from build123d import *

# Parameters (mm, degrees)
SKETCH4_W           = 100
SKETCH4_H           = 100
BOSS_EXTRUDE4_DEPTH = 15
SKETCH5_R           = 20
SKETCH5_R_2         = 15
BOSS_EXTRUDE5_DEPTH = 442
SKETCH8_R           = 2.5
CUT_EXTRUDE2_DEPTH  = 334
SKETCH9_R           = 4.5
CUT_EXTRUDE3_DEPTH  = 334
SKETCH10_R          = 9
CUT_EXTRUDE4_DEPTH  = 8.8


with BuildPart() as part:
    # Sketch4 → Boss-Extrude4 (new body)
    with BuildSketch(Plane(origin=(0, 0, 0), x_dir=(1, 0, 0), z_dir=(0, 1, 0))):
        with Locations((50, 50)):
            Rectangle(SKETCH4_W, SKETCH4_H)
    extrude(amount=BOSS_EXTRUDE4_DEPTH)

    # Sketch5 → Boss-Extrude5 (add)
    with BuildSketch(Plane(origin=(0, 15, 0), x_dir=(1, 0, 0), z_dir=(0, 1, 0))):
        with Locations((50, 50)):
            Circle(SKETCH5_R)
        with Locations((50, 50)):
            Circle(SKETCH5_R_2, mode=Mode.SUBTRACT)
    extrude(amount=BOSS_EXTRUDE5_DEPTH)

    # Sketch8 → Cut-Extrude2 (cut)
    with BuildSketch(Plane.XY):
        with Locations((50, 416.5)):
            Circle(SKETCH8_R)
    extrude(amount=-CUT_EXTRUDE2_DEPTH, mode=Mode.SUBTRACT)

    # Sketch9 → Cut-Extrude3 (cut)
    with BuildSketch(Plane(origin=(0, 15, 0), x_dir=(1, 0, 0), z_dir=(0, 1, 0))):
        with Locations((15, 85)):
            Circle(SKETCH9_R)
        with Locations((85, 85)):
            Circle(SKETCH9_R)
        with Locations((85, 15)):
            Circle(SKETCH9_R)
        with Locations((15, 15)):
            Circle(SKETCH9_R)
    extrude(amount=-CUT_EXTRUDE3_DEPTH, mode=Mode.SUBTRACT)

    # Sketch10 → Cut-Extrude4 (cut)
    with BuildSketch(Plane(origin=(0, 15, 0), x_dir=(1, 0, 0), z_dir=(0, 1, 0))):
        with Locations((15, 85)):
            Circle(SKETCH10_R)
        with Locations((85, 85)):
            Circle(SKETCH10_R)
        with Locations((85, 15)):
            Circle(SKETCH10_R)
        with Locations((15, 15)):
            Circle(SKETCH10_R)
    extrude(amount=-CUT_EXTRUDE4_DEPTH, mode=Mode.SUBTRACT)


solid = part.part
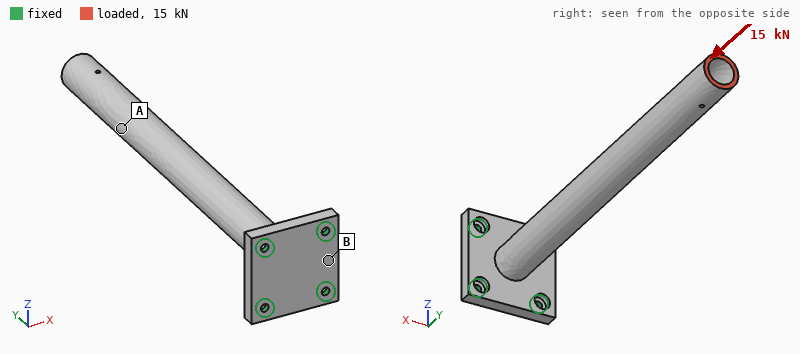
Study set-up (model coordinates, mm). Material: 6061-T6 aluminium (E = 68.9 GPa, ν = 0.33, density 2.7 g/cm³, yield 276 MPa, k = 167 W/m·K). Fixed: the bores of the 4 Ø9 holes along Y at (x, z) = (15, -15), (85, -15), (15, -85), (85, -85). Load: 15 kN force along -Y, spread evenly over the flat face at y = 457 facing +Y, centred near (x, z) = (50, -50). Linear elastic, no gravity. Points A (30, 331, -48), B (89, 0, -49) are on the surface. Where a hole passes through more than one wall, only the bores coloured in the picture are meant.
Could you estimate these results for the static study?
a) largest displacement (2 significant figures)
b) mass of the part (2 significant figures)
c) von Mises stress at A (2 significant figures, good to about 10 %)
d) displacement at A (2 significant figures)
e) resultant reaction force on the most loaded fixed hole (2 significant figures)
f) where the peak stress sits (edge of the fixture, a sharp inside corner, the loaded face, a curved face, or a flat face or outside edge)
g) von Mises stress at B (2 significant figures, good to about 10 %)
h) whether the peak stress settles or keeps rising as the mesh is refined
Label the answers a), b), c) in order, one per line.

a) 0.22 mm
b) 1.0 kg
c) 27 MPa
d) 0.16 mm
e) 5.2 kN
f) edge of the fixture
g) 17 MPa
h) keeps rising
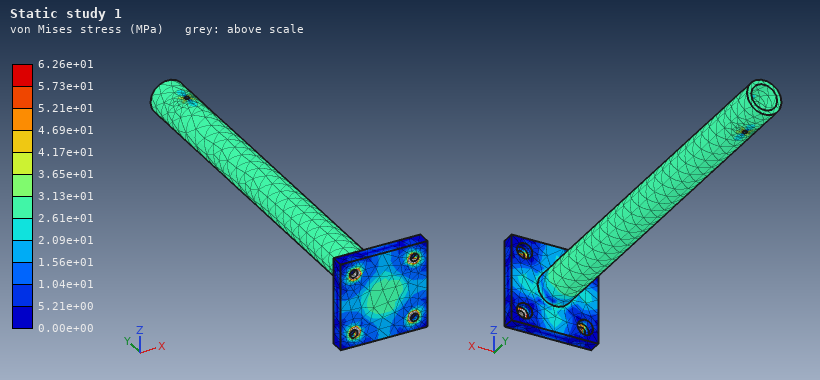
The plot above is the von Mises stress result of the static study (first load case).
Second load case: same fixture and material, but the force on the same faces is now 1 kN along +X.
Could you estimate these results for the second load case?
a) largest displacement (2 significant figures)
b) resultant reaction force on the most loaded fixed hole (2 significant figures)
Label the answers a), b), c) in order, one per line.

a) 5.6 mm
b) 4.0 kN
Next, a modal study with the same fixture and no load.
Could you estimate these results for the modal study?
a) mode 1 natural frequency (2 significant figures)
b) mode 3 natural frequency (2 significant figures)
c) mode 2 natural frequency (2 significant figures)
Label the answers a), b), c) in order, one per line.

a) 160 Hz
b) 990 Hz
c) 160 Hz
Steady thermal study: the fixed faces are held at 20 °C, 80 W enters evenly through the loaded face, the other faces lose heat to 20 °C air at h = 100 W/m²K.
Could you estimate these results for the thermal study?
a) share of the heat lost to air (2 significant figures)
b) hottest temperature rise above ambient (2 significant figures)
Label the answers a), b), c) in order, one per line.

a) 100 %
b) 57 K
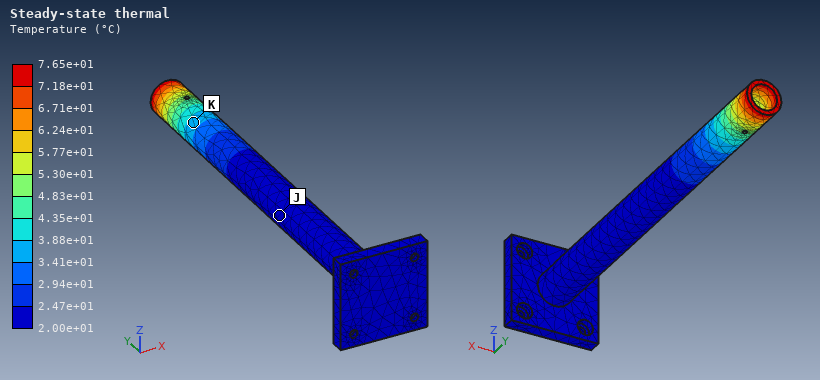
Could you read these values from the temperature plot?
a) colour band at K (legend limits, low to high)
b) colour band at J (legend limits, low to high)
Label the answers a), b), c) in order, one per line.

a) 3.41e+01 to 3.88e+01 °C
b) 2.00e+01 to 2.47e+01 °C
